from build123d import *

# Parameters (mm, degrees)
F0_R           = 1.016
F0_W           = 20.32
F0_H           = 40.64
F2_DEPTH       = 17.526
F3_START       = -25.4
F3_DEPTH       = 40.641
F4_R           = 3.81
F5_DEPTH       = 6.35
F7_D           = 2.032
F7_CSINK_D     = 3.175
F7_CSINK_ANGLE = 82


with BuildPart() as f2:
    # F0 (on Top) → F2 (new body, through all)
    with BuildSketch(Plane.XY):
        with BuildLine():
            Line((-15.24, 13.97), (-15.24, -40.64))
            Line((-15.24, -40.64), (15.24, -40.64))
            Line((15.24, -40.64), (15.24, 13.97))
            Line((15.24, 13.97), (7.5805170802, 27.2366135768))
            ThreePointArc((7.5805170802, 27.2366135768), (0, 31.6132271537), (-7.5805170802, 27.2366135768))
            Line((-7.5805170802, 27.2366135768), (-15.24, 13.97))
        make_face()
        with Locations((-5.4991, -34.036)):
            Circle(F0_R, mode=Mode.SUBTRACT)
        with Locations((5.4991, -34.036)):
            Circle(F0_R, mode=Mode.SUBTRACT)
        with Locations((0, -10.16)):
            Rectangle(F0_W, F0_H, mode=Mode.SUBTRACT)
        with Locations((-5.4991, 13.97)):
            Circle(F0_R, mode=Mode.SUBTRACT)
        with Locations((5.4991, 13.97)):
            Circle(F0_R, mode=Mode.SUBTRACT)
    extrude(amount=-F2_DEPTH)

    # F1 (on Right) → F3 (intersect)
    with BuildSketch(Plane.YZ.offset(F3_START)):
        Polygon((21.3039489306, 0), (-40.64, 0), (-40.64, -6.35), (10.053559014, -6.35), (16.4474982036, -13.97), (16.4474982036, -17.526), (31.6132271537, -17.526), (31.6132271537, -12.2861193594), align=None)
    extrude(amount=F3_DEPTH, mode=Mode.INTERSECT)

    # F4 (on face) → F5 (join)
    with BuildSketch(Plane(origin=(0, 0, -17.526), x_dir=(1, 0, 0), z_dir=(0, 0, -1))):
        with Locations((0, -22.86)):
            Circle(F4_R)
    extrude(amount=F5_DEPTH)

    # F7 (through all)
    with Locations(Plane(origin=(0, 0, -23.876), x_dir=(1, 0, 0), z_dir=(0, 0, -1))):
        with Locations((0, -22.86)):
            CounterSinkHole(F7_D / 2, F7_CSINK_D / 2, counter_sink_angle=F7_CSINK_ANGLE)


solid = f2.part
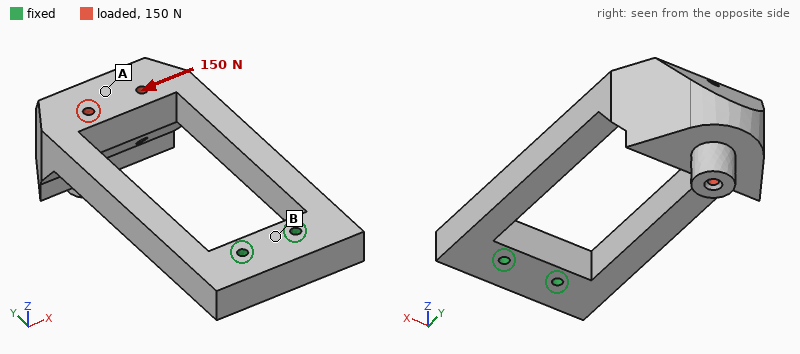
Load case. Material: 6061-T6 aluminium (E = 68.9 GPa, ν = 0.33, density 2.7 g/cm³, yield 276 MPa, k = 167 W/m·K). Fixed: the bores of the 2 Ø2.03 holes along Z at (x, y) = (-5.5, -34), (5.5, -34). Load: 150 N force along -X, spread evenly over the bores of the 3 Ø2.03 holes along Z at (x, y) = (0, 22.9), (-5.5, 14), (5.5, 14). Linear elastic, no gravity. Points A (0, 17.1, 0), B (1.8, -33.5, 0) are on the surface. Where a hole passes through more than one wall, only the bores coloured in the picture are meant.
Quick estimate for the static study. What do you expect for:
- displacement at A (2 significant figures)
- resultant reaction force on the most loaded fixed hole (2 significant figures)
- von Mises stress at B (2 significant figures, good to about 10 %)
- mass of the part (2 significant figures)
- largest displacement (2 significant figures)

0.16 mm
570 N
9.5 MPa
29 g
0.22 mm
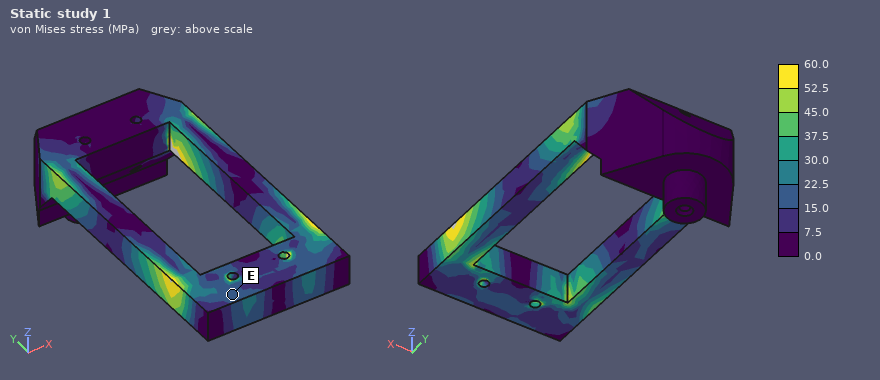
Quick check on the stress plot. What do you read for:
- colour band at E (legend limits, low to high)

15.0 to 22.5 MPa
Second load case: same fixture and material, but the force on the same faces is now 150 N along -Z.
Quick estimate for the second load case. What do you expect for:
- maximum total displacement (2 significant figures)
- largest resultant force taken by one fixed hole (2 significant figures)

0.81 mm
75 N
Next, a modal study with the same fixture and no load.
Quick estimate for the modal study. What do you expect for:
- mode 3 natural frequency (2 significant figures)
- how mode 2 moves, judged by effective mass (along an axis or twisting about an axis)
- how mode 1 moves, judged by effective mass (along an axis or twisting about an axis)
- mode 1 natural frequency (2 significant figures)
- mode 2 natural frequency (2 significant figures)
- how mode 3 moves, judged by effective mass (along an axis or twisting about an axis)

2400 Hz
along X
along Z
580 Hz
1000 Hz
twisting about Y
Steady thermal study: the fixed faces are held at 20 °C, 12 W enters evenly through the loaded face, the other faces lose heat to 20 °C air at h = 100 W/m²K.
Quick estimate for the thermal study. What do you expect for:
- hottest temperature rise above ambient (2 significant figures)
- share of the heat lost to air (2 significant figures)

26 K
63 %
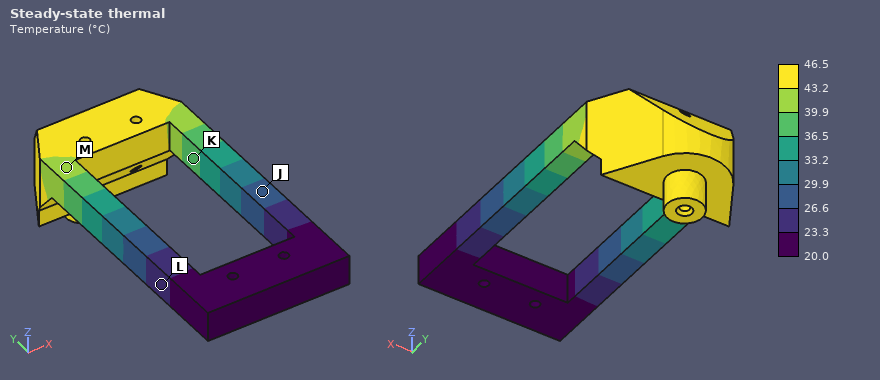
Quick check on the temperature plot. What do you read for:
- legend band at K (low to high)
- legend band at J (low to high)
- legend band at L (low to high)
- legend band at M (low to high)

36.5 to 39.9 °C
26.6 to 29.9 °C
23.3 to 26.6 °C
39.9 to 43.2 °C
